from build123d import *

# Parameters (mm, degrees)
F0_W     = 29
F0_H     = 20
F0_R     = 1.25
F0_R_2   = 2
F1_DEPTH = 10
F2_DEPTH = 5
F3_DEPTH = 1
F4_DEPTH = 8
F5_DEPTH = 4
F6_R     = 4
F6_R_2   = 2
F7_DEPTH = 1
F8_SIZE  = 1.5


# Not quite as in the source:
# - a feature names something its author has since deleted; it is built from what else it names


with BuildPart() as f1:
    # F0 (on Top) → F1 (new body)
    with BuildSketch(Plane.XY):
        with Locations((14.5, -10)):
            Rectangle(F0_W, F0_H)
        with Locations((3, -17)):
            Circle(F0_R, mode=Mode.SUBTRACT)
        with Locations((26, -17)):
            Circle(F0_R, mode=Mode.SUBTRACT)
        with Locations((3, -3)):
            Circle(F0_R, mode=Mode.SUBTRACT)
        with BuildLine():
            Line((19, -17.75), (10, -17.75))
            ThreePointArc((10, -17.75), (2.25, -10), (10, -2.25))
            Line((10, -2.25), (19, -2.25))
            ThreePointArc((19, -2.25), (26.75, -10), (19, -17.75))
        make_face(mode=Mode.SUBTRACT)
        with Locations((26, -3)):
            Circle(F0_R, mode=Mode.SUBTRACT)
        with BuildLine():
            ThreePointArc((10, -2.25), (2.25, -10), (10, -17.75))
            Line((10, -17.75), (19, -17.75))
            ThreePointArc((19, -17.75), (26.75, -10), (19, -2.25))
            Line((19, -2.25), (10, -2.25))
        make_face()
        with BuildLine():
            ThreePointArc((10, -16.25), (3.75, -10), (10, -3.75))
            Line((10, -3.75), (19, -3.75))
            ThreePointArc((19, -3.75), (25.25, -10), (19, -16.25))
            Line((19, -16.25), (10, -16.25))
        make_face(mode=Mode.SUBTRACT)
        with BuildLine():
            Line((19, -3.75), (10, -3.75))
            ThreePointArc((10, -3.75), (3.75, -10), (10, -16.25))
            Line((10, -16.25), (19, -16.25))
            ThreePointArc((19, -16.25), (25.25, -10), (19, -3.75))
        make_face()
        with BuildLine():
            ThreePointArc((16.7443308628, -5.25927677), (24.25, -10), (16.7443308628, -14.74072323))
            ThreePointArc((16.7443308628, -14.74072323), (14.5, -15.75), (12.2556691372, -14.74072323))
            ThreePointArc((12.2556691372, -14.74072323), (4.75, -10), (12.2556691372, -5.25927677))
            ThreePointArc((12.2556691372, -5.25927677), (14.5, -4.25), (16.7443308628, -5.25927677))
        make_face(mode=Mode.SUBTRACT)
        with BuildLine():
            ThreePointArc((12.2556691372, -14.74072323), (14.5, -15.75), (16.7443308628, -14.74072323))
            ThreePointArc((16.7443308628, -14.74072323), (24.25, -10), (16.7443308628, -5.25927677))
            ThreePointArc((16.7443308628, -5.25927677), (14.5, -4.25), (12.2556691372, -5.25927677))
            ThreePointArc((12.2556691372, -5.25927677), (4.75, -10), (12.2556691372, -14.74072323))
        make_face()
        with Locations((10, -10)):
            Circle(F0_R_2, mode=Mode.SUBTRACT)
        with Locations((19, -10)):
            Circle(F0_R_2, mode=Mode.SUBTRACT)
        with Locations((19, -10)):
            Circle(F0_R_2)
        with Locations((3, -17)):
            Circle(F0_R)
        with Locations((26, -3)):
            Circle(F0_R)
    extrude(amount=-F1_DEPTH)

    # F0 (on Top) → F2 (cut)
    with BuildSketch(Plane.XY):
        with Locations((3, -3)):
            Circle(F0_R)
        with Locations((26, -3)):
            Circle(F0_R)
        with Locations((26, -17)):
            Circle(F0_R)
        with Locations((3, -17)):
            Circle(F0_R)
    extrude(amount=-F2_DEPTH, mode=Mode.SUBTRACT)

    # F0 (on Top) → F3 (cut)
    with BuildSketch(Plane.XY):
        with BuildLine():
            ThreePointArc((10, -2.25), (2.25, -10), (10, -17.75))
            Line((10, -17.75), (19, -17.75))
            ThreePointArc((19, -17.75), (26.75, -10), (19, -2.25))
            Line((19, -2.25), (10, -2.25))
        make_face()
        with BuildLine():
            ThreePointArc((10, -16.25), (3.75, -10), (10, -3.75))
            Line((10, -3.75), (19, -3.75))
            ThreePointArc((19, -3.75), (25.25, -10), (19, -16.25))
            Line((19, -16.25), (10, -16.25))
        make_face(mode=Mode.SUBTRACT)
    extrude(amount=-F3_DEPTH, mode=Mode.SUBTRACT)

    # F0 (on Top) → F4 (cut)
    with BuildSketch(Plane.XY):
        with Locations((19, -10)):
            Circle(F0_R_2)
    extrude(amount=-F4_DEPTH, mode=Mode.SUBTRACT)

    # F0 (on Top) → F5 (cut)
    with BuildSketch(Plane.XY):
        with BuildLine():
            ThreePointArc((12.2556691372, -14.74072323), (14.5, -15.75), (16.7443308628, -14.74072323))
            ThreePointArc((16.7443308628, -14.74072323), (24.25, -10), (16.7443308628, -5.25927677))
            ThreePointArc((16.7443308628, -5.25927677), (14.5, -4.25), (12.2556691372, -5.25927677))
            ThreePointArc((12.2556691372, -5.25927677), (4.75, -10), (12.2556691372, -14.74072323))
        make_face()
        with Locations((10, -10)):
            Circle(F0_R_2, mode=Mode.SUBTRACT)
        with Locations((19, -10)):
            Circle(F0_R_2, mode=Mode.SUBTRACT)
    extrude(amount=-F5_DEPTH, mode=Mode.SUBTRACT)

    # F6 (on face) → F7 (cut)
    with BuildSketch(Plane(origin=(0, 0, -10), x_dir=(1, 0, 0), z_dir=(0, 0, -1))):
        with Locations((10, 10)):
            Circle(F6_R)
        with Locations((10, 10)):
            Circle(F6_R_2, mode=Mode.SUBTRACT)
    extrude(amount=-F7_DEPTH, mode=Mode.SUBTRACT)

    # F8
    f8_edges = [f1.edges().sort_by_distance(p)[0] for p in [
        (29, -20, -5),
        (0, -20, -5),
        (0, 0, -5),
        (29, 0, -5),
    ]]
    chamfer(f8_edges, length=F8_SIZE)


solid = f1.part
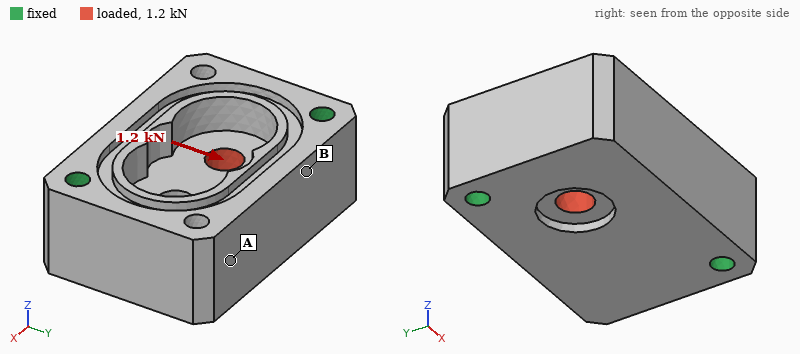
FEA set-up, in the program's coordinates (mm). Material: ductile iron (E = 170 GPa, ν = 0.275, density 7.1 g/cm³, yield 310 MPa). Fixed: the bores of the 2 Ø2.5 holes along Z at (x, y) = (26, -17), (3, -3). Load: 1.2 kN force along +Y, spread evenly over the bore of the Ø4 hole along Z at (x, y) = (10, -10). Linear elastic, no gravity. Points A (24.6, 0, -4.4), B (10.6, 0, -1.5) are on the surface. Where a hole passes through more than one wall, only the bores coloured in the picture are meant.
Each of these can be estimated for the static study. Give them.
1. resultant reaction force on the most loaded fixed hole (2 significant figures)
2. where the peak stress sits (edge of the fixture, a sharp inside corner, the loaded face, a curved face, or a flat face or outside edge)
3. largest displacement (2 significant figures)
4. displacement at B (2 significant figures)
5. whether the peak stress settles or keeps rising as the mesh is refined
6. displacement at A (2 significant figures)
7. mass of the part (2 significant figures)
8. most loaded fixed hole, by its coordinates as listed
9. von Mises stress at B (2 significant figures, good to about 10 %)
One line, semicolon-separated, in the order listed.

830 N; edge of the fixture; 1.5 µm; 0.69 µm; keeps rising; 0.77 µm; 33 g; (3, -3); 9.6 MPa
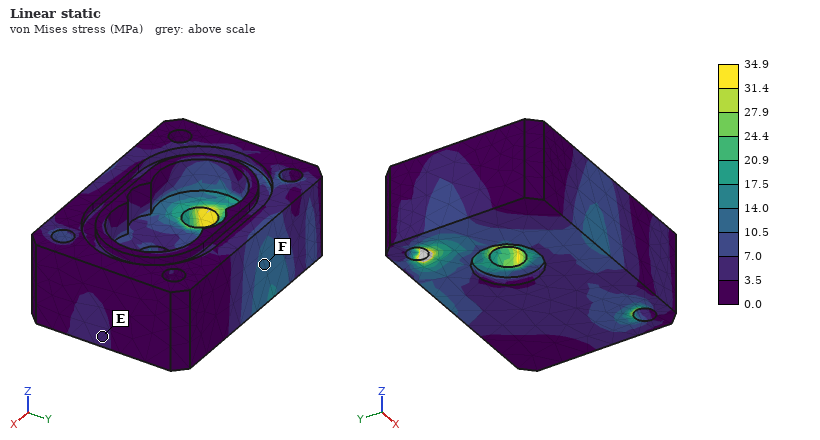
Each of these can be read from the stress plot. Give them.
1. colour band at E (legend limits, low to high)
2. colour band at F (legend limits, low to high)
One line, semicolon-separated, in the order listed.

3.5 to 7.0 MPa; 10.5 to 14.0 MPa
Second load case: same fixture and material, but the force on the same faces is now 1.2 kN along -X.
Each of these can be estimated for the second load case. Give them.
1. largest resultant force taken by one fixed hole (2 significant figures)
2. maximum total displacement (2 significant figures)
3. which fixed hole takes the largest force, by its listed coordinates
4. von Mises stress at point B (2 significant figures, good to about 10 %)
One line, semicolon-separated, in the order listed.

680 N; 1.2 µm; (3, -3); 6.1 MPa
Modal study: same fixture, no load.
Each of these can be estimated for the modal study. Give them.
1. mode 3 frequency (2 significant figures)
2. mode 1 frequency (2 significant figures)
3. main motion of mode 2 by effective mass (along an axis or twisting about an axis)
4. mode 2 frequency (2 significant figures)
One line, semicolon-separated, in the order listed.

38 kHz; 22 kHz; along Z; 25 kHz
